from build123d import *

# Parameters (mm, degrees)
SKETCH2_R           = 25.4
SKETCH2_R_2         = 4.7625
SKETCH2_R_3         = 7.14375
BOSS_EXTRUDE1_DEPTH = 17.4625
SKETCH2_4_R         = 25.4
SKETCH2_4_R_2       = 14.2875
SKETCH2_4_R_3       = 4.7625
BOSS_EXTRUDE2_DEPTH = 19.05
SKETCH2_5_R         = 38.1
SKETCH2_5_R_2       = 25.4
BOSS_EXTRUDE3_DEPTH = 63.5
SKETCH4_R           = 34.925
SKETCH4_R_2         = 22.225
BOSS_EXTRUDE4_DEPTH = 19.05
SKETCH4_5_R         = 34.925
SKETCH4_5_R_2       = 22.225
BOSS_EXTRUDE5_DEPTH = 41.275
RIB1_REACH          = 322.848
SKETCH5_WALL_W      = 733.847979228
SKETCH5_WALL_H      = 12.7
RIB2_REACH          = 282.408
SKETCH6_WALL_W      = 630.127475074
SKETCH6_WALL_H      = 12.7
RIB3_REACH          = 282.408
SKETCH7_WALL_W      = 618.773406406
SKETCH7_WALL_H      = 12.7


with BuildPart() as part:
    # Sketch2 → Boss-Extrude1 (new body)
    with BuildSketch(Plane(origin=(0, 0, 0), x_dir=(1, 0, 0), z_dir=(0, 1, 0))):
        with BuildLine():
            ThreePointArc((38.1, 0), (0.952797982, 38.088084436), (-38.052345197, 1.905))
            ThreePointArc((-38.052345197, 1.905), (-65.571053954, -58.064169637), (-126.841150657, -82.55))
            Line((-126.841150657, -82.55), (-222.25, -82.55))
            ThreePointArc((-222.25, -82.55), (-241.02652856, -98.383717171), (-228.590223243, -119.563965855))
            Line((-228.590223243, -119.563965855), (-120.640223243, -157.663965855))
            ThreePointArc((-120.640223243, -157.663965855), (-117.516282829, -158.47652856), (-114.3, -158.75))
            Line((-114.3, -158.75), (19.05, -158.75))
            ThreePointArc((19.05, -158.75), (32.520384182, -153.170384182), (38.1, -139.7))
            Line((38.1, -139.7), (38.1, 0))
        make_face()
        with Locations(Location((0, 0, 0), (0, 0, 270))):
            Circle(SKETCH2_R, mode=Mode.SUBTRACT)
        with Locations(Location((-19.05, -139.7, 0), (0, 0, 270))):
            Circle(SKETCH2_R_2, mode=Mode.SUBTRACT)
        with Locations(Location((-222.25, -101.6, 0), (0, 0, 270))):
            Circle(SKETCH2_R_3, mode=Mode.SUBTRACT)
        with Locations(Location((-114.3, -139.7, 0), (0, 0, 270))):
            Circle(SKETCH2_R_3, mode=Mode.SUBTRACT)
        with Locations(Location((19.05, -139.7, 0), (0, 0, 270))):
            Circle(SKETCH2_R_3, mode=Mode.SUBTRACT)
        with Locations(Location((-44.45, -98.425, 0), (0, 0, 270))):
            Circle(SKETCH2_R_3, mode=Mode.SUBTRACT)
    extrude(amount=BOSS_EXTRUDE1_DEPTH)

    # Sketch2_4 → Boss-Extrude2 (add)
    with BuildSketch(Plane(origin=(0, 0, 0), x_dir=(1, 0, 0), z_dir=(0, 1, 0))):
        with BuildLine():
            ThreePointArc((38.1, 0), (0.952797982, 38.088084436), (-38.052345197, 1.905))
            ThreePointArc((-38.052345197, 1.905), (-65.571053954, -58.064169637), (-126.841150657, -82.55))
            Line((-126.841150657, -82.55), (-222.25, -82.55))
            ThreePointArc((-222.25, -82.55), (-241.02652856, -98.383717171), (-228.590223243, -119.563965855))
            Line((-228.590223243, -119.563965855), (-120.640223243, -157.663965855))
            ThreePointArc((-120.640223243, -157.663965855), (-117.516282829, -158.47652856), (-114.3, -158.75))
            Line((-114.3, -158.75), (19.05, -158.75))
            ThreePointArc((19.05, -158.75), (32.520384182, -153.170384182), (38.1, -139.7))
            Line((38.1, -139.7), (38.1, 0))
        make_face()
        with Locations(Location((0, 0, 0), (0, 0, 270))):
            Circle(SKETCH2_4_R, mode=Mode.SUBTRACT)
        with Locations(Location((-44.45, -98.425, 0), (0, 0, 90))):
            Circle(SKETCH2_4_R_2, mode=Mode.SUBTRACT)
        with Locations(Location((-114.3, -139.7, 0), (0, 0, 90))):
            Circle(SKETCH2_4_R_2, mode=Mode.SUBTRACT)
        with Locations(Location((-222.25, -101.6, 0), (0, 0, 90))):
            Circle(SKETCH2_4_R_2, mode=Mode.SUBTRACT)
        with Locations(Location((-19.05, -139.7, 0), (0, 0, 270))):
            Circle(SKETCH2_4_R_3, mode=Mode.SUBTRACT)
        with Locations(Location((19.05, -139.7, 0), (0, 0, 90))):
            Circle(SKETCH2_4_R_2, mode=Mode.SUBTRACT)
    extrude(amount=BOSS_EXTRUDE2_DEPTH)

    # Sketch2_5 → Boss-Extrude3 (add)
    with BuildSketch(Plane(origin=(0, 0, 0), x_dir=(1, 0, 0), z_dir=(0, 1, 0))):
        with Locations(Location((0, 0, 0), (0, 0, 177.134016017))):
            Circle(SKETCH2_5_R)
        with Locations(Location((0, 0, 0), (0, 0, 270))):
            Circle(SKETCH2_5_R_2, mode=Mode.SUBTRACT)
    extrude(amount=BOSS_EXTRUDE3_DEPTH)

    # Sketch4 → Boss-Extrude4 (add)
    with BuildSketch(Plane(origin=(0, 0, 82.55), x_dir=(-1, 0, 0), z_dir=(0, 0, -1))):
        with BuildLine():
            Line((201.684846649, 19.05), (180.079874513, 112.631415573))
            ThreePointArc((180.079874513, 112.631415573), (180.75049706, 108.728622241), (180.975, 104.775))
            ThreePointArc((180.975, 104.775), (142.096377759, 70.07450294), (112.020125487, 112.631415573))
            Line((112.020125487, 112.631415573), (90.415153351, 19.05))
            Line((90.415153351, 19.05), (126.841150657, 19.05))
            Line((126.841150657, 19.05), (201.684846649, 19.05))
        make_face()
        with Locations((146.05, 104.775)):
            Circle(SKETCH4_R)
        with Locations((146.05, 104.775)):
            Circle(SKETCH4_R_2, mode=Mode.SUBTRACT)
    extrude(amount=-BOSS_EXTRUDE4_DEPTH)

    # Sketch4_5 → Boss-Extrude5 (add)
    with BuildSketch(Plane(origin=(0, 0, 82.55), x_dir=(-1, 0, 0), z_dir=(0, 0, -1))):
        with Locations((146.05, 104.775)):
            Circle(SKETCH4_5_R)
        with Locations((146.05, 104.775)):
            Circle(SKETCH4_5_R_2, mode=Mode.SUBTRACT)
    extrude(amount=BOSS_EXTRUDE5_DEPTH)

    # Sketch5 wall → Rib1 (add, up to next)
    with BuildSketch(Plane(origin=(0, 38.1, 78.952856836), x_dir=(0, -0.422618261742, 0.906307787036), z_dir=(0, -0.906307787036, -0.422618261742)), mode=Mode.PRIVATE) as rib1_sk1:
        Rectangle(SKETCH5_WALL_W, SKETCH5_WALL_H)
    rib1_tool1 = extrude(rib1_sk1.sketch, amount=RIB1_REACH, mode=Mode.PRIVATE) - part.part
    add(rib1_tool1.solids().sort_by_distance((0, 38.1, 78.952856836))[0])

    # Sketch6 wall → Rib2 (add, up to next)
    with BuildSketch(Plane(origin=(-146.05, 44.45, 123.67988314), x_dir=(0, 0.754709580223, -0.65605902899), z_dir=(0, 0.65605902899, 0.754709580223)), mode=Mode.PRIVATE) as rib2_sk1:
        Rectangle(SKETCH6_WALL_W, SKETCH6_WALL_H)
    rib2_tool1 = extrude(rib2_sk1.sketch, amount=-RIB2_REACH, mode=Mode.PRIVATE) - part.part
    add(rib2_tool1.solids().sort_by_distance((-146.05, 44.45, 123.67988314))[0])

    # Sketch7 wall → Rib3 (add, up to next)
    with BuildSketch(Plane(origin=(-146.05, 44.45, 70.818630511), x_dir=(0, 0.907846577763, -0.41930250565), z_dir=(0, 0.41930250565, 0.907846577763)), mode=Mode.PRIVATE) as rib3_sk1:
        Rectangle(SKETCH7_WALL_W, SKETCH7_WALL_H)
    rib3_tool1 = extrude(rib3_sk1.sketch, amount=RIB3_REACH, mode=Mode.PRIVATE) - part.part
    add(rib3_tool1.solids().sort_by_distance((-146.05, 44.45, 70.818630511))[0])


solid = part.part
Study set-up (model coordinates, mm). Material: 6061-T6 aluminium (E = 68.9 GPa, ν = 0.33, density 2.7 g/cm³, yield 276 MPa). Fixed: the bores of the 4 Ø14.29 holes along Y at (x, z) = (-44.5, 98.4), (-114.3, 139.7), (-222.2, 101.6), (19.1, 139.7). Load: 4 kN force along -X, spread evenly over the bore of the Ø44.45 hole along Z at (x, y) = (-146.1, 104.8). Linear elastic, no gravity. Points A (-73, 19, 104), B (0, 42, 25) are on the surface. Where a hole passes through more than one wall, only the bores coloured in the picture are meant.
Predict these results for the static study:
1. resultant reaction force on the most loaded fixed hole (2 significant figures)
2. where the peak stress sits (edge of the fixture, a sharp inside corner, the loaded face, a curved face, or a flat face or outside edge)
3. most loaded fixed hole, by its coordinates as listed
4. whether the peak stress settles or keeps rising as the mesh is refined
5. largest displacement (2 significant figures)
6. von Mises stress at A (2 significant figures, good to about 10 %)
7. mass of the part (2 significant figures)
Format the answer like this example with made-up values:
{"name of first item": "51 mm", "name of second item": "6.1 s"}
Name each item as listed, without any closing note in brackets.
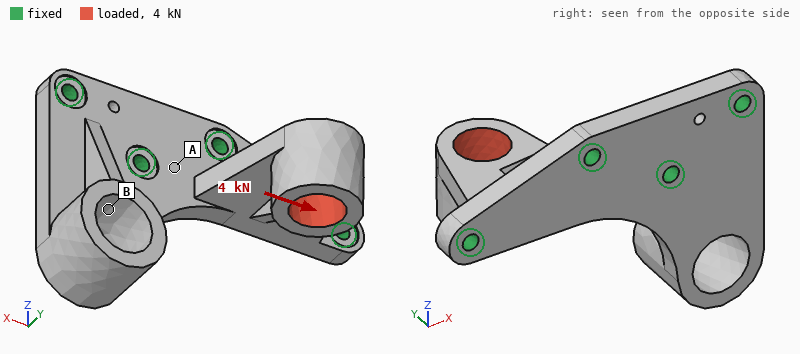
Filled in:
{"resultant reaction force on the most loaded fixed hole": "3.8 kN", "where the peak stress sits": "edge of the fixture", "most loaded fixed hole, by its coordinates as listed": "(-222.2, 101.6)", "whether the peak stress settles or keeps rising as the mesh is refined": "keeps rising", "largest displacement": "83 µm", "von Mises stress at A": "4.6 MPa", "mass of the part": "2.4 kg"}
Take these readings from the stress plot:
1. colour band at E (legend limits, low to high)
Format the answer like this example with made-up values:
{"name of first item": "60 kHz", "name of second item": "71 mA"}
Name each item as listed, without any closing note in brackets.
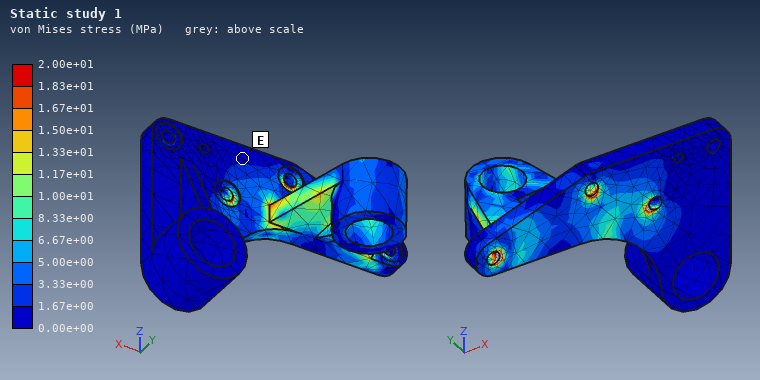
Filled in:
{"colour band at E": "0.00e+00 to 1.67e+00 MPa"}
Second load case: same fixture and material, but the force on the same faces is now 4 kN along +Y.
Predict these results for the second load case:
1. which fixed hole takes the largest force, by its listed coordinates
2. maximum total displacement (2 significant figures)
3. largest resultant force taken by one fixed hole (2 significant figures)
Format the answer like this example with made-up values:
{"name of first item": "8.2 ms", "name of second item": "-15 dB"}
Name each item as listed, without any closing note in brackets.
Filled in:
{"which fixed hole takes the largest force, by its listed coordinates": "(-222.2, 101.6)", "maximum total displacement": "0.15 mm", "largest resultant force taken by one fixed hole": "2.6 kN"}
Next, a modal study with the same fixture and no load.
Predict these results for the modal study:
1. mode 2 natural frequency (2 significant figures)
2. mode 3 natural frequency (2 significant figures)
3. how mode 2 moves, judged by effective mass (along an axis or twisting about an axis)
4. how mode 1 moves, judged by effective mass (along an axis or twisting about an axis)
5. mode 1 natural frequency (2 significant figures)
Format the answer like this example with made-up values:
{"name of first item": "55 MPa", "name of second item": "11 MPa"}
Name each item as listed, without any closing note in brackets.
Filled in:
{"mode 2 natural frequency": "940 Hz", "mode 3 natural frequency": "1800 Hz", "how mode 2 moves, judged by effective mass": "along Z", "how mode 1 moves, judged by effective mass": "along Y", "mode 1 natural frequency": "720 Hz"}
